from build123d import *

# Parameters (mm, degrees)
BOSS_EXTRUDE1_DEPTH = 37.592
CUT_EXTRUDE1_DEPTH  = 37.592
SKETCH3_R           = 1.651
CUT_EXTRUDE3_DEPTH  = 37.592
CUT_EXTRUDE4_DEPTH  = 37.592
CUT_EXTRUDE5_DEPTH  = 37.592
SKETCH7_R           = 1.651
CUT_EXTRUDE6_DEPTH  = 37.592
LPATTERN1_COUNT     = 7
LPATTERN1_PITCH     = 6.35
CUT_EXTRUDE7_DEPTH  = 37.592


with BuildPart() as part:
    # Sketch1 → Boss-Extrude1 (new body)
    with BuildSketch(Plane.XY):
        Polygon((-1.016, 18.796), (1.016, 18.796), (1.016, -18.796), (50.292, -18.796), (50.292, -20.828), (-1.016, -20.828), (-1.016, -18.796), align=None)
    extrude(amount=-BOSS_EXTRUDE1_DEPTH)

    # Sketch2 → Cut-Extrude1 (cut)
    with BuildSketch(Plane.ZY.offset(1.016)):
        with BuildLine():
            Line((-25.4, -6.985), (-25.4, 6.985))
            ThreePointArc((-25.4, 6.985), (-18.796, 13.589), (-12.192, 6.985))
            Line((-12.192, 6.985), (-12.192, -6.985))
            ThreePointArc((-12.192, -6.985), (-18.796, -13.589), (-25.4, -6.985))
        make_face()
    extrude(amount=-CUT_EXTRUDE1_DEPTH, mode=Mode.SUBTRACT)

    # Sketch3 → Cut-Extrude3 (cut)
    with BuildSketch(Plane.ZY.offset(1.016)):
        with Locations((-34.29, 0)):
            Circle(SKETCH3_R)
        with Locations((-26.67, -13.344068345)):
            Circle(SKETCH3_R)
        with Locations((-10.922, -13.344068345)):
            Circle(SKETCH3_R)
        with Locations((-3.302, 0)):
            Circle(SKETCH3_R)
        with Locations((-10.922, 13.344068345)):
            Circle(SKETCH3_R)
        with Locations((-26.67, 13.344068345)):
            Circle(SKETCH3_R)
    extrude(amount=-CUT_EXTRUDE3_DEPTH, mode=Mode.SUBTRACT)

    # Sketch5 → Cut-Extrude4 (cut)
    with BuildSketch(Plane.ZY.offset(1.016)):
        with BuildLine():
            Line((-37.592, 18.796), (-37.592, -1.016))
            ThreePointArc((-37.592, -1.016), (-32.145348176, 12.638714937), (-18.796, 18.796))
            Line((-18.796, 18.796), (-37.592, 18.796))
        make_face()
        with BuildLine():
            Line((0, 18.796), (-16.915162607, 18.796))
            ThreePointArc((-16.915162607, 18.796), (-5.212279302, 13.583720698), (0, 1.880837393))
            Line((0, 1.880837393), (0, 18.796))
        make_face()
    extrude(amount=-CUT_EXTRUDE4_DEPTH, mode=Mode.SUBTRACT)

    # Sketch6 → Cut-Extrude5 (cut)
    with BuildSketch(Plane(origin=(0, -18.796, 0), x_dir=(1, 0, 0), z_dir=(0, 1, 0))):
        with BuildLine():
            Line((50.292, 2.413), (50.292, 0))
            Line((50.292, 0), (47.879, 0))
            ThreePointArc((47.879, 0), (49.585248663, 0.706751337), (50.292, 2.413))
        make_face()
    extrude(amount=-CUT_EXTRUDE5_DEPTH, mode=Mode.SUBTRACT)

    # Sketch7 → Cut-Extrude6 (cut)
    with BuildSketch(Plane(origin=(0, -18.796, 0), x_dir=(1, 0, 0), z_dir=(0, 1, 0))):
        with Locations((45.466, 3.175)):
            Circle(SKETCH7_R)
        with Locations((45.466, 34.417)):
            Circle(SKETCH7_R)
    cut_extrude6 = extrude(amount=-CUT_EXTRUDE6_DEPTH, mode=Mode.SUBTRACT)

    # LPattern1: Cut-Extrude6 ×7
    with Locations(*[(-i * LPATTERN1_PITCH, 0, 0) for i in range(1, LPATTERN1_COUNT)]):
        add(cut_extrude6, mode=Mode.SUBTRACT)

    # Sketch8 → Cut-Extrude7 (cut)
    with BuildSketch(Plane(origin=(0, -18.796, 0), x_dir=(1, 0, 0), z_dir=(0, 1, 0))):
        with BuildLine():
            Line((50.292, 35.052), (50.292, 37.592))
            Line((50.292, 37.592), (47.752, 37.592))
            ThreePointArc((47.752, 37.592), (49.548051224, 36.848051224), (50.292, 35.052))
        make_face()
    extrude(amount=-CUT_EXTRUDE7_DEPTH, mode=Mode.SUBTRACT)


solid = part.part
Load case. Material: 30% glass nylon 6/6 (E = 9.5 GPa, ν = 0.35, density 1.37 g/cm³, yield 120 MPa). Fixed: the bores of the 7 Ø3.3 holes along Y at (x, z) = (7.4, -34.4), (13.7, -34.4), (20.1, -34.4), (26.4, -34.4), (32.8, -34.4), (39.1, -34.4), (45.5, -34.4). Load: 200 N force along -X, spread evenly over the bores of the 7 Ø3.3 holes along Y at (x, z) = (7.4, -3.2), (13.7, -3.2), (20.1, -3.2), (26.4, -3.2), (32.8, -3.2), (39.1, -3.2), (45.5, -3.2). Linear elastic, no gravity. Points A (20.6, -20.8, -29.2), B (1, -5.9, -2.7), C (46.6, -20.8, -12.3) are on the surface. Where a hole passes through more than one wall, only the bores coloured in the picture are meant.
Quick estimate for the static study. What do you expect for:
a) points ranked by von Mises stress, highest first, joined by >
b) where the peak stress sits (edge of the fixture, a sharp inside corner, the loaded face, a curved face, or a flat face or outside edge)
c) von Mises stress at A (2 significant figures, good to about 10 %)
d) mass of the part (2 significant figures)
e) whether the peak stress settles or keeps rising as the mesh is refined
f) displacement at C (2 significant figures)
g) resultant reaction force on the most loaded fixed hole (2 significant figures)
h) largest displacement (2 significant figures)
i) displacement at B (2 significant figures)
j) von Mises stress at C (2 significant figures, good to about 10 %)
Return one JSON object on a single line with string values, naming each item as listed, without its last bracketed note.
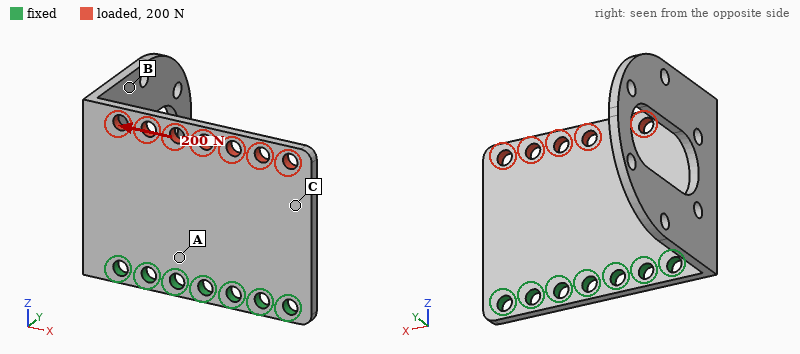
{"points ranked by von Mises stress, highest first, joined by >": "A > C > B", "where the peak stress sits": "edge of the fixture", "von Mises stress at A": "4.9 MPa", "mass of the part": "7.5 g", "whether the peak stress settles or keeps rising as the mesh is refined": "keeps rising", "displacement at C": "24 µm", "resultant reaction force on the most loaded fixed hole": "130 N", "largest displacement": "41 µm", "displacement at B": "34 µm", "von Mises stress at C": "2.4 MPa"}
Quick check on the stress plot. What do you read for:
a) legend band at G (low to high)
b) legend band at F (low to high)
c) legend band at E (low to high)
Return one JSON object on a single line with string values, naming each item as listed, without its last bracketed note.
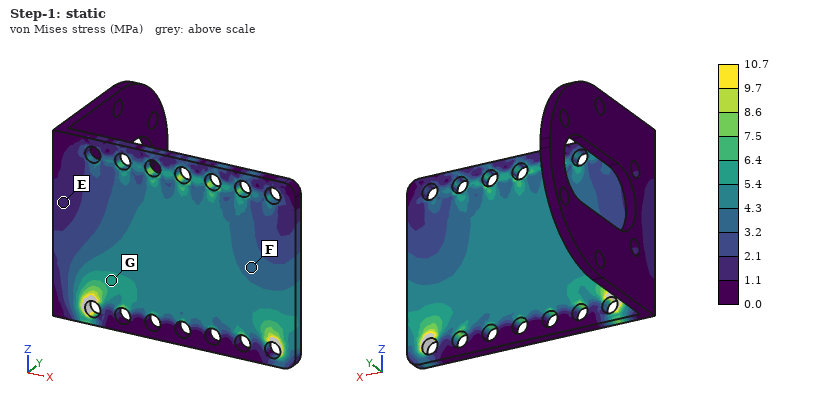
{"legend band at G": "5.4 to 6.4 MPa", "legend band at F": "3.2 to 4.3 MPa", "legend band at E": "1.1 to 2.1 MPa"}
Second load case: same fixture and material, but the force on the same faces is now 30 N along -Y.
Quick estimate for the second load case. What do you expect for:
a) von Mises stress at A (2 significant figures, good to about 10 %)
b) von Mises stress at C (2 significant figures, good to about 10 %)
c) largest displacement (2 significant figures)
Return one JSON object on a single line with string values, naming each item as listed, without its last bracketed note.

{"von Mises stress at A": "16 MPa", "von Mises stress at C": "6.7 MPa", "largest displacement": "0.76 mm"}
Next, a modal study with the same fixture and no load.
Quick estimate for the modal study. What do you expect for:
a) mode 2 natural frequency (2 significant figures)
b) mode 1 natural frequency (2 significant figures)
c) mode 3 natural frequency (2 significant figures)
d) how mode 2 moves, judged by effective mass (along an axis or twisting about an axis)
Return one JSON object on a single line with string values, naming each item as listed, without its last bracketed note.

{"mode 2 natural frequency": "640 Hz", "mode 1 natural frequency": "480 Hz", "mode 3 natural frequency": "1100 Hz", "how mode 2 moves, judged by effective mass": "along Y"}
